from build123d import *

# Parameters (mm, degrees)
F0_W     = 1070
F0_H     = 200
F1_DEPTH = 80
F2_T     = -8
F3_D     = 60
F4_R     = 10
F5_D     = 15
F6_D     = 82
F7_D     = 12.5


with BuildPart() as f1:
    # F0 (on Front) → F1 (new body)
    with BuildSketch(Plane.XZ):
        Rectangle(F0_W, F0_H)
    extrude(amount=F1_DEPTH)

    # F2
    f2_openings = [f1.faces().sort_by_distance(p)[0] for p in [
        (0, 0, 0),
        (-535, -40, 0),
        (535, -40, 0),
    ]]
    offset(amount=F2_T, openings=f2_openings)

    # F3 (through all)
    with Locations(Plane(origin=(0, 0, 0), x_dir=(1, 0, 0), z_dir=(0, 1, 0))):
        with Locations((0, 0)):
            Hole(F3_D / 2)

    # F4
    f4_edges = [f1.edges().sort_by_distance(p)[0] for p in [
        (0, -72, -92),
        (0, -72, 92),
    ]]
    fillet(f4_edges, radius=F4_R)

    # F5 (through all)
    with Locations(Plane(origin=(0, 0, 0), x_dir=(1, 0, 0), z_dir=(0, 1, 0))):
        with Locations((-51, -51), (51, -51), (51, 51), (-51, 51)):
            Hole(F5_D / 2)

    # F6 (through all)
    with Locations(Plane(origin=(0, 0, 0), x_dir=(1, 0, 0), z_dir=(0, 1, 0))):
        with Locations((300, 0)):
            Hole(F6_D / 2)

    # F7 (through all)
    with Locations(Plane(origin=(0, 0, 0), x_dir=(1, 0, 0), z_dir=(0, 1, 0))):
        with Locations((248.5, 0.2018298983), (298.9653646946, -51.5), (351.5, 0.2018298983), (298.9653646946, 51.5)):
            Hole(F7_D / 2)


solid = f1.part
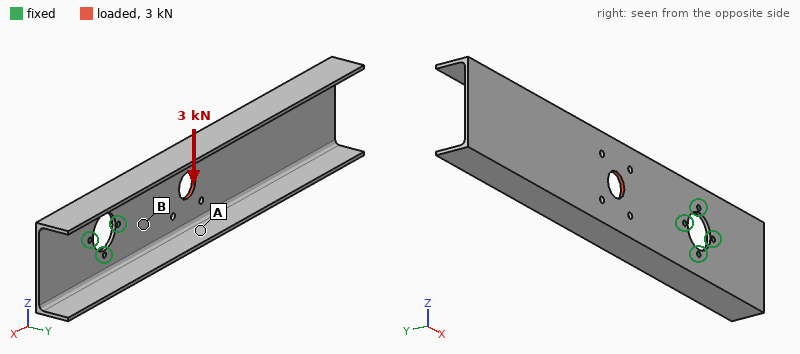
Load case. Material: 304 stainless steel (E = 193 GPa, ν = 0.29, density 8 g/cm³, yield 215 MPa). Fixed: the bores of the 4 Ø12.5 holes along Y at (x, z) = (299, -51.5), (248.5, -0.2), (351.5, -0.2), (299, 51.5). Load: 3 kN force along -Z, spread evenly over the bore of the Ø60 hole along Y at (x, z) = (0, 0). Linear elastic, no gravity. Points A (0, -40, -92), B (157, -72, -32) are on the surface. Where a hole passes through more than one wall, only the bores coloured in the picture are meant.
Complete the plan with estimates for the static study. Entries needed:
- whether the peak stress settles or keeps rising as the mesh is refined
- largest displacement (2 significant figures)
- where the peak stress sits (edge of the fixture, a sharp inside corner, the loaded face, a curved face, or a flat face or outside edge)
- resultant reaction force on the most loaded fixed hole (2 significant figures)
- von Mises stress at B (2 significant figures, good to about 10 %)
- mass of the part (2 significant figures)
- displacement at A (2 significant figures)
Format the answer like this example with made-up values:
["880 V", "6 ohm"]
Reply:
["keeps rising", "0.11 mm", "edge of the fixture", "4.9 kN", "4.4 MPa", "23 kg", "0.034 mm"]
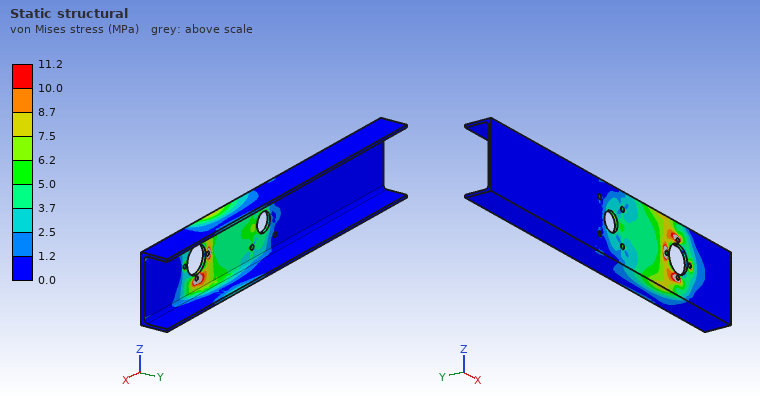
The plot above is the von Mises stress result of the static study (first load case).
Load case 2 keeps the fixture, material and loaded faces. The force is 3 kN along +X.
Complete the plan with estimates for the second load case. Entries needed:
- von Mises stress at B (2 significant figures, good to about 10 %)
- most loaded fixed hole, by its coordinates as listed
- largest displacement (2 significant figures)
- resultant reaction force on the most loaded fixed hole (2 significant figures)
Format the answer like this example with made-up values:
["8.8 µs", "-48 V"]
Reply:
["1.7 MPa", "(248.5, -0.2)", "29 µm", "1.2 kN"]
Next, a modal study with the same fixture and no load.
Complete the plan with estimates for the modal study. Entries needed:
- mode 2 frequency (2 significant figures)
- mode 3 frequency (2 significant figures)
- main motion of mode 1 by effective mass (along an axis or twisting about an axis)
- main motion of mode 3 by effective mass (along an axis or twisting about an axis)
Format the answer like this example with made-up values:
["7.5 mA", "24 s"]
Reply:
["65 Hz", "180 Hz", "along Y", "along Z"]
